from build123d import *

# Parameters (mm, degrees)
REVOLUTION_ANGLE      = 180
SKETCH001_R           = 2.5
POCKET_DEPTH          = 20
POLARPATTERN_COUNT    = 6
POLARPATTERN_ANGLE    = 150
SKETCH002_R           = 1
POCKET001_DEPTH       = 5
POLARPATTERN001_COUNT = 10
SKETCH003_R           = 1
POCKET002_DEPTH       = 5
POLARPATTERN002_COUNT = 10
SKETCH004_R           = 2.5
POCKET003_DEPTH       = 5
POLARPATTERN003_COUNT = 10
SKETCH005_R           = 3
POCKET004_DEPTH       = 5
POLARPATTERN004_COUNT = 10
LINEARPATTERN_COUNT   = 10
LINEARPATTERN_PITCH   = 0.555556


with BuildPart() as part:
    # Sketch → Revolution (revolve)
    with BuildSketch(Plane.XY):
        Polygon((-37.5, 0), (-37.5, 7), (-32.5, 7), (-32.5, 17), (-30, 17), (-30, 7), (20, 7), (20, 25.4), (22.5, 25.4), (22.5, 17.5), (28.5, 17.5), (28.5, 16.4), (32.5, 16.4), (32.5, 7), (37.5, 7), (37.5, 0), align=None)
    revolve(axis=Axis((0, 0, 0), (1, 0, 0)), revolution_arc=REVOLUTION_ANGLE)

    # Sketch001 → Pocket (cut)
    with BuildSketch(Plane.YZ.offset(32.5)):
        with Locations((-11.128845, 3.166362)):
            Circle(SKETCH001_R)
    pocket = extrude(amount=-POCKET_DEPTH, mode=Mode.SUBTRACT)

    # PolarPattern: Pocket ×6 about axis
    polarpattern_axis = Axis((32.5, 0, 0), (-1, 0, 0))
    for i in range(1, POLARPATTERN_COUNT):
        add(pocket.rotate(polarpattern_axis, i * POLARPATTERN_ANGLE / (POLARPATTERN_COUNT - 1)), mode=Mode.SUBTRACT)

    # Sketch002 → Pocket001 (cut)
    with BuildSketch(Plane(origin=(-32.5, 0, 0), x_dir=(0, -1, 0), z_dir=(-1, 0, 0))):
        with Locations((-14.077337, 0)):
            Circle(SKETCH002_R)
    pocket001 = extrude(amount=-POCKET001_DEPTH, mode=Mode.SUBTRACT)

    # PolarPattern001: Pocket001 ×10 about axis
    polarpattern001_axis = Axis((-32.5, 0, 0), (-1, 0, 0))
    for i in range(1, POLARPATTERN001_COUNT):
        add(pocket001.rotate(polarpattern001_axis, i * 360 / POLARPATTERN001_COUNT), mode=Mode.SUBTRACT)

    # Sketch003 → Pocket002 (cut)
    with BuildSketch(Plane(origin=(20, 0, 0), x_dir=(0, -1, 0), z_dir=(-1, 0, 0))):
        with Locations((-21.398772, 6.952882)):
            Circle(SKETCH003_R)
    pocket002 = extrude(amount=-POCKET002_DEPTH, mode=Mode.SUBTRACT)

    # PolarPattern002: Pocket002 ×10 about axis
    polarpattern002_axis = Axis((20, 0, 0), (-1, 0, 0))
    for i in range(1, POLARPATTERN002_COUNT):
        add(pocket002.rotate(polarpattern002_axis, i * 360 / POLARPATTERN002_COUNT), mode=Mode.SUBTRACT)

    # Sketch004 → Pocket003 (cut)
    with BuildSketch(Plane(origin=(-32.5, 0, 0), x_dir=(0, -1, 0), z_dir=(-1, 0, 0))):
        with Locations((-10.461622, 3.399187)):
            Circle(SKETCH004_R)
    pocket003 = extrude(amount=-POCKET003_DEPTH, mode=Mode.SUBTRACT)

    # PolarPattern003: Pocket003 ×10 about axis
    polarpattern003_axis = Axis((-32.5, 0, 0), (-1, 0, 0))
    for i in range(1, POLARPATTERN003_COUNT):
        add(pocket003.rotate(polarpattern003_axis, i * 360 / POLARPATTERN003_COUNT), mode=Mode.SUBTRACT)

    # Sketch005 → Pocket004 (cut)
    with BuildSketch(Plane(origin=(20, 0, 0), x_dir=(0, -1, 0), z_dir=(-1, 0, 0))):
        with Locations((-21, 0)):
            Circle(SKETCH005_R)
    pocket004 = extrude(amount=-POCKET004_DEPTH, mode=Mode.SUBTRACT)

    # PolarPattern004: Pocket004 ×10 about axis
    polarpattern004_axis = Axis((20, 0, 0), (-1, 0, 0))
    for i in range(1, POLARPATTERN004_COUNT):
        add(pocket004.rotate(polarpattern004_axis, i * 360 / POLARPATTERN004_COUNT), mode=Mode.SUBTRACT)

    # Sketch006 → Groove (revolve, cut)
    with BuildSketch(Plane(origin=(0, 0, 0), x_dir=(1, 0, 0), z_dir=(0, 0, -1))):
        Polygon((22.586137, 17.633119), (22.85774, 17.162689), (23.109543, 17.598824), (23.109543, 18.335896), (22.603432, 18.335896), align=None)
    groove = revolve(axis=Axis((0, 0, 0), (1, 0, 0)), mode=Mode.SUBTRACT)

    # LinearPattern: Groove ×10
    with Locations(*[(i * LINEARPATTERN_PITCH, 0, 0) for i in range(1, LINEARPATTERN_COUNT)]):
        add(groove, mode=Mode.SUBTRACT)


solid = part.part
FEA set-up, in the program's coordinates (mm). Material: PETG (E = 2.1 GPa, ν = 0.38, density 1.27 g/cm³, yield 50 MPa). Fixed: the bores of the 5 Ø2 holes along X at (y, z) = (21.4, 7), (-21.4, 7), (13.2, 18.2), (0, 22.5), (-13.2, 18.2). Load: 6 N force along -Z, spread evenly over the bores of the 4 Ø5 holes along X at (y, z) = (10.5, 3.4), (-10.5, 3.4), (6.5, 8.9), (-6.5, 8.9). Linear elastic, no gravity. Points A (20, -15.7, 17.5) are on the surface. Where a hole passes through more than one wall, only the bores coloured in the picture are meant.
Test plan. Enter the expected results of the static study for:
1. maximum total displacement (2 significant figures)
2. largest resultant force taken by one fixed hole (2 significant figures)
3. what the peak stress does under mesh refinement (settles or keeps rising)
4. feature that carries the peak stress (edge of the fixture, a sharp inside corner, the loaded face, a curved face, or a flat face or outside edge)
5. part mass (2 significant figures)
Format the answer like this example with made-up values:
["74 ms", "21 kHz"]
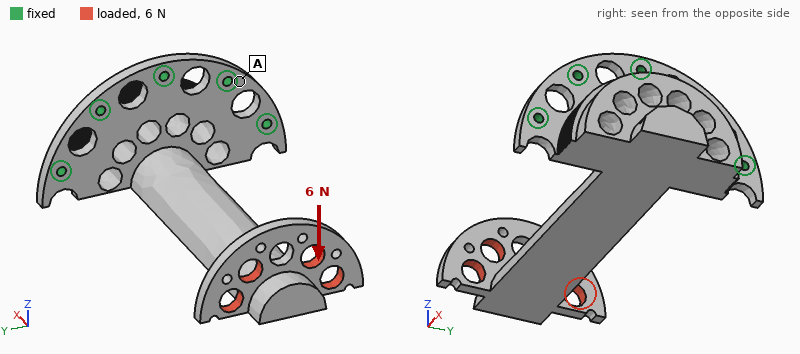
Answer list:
["0.89 mm", "14 N", "keeps rising", "edge of the fixture", "14 g"]
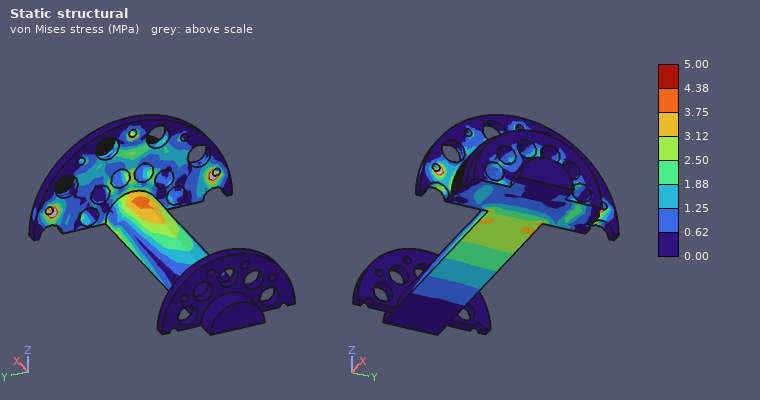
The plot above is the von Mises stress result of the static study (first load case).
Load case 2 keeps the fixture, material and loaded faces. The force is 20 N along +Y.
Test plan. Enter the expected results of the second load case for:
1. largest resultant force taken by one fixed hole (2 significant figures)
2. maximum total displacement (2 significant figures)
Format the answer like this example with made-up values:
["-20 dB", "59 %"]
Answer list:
["22 N", "0.91 mm"]
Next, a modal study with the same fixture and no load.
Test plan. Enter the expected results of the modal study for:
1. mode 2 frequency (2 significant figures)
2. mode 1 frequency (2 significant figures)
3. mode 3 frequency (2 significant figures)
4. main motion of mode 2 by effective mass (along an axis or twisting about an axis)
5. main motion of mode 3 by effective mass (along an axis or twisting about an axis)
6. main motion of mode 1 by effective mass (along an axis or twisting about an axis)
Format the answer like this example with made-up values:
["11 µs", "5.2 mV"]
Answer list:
["460 Hz", "260 Hz", "1200 Hz", "along Y", "along X", "along Z"]
